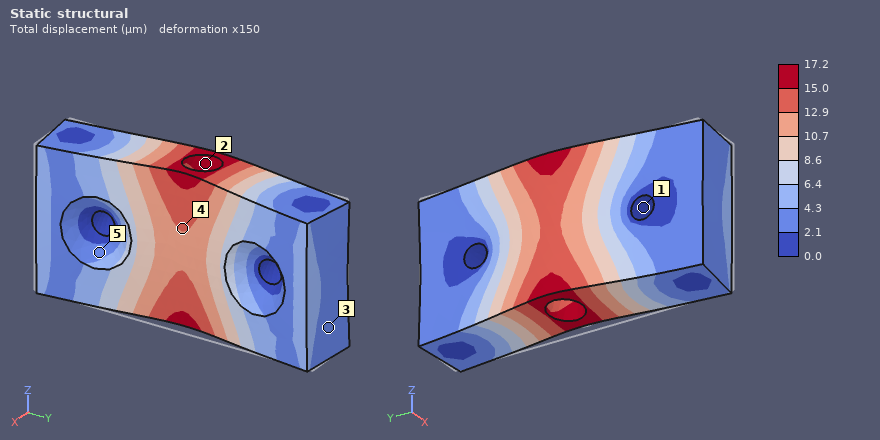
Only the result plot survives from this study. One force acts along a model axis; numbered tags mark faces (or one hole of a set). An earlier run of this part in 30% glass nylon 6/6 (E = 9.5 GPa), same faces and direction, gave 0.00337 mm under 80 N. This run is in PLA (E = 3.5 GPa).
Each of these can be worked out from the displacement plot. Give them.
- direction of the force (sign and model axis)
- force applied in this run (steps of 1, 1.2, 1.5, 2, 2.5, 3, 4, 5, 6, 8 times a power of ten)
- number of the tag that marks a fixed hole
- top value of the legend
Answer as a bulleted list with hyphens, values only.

- -X
- 150 N
- 1
- 17.2 µm
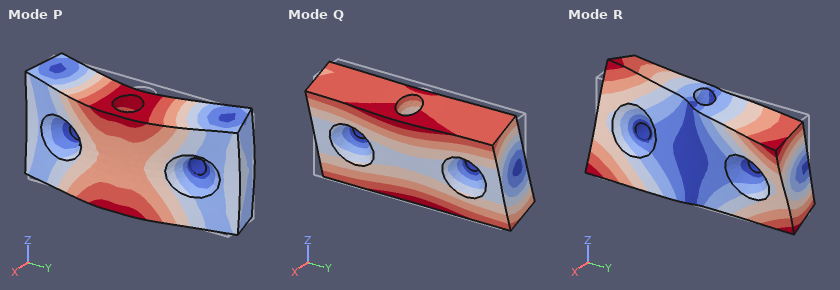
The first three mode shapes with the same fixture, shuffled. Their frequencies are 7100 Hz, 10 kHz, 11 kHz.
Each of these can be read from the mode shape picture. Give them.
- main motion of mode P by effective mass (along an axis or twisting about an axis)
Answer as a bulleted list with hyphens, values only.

- along X
